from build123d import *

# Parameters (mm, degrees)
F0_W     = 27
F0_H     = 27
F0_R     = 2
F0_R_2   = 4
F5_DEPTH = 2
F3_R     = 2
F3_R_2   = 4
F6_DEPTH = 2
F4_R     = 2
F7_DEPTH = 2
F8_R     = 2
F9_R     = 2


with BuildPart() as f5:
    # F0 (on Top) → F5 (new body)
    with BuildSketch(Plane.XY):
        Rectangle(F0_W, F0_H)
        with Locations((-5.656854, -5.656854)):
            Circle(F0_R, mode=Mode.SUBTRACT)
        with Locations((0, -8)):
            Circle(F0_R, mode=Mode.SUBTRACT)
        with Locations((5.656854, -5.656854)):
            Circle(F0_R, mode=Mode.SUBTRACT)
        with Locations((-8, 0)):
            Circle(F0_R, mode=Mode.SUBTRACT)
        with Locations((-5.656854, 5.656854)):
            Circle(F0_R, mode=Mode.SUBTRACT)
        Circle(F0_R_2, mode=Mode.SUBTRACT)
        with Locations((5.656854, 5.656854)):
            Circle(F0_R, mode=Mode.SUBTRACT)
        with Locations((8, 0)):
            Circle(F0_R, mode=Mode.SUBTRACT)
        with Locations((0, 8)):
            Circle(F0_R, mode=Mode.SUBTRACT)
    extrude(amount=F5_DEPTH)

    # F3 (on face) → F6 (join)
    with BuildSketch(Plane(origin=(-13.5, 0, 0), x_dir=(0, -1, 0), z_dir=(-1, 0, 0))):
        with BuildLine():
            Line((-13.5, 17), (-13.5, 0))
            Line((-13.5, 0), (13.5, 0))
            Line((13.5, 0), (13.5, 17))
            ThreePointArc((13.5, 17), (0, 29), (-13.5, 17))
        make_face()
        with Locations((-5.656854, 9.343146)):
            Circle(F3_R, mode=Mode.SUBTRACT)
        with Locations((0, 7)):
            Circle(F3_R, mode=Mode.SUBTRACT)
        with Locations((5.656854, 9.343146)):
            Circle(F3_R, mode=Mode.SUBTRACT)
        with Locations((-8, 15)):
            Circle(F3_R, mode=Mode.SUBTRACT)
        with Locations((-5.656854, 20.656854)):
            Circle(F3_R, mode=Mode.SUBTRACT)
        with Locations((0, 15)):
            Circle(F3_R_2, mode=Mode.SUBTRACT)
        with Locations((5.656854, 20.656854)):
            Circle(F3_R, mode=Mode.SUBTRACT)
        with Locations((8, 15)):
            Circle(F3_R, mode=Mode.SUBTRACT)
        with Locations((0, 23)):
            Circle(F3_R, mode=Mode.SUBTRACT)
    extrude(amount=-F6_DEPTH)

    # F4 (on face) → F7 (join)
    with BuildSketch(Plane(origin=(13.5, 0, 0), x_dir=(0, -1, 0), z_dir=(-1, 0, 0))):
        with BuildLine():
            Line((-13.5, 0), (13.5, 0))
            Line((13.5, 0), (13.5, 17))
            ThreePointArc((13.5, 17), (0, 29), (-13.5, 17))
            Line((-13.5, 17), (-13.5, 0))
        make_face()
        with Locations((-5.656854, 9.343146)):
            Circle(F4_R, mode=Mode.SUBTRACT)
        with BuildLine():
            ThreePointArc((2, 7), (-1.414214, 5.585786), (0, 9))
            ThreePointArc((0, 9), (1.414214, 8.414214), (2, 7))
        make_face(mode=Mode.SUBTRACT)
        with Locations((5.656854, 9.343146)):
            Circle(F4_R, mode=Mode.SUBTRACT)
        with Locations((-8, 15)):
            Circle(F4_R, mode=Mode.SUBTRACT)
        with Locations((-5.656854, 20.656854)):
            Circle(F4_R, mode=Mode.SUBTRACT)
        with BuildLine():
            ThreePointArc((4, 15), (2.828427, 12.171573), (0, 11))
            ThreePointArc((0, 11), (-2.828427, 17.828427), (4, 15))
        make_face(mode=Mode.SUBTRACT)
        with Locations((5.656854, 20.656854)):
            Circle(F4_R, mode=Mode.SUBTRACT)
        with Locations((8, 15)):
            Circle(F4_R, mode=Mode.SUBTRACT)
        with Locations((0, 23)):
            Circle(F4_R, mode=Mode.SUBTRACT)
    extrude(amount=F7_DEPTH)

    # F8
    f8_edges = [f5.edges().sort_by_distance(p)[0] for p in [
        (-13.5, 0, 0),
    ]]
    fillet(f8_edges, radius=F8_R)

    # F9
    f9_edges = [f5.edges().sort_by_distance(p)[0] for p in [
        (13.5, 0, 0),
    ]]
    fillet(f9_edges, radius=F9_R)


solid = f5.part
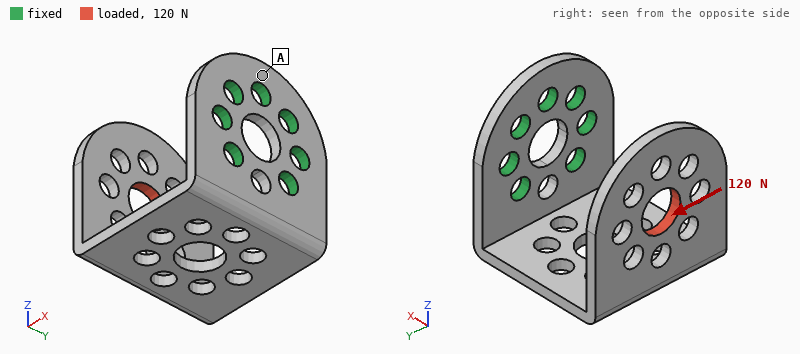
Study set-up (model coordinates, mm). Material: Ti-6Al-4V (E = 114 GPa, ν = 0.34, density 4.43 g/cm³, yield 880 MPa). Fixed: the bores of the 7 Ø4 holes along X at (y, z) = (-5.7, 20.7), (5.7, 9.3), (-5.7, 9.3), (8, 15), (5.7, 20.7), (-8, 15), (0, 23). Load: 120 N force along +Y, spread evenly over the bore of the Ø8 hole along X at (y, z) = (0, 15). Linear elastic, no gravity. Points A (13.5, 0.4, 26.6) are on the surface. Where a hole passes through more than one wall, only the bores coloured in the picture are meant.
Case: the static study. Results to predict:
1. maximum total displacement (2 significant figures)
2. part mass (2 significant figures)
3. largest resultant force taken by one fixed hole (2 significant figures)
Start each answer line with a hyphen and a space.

- 0.56 mm
- 14 g
- 230 N
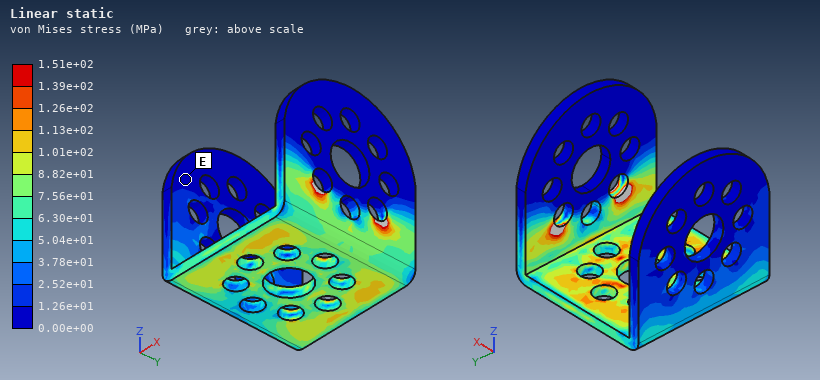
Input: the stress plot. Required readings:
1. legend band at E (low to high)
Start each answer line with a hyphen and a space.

- 0.00e+00 to 1.26e+01 MPa
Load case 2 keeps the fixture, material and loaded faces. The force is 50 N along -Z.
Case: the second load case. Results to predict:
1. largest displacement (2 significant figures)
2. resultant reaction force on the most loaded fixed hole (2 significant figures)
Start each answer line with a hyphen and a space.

- 0.53 mm
- 35 N
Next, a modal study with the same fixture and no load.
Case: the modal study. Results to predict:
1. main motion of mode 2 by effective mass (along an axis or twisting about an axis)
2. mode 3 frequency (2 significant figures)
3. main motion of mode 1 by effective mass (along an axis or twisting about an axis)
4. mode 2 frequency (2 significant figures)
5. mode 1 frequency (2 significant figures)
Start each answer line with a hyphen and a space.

- along Y
- 2000 Hz
- along Z
- 1200 Hz
- 690 Hz
